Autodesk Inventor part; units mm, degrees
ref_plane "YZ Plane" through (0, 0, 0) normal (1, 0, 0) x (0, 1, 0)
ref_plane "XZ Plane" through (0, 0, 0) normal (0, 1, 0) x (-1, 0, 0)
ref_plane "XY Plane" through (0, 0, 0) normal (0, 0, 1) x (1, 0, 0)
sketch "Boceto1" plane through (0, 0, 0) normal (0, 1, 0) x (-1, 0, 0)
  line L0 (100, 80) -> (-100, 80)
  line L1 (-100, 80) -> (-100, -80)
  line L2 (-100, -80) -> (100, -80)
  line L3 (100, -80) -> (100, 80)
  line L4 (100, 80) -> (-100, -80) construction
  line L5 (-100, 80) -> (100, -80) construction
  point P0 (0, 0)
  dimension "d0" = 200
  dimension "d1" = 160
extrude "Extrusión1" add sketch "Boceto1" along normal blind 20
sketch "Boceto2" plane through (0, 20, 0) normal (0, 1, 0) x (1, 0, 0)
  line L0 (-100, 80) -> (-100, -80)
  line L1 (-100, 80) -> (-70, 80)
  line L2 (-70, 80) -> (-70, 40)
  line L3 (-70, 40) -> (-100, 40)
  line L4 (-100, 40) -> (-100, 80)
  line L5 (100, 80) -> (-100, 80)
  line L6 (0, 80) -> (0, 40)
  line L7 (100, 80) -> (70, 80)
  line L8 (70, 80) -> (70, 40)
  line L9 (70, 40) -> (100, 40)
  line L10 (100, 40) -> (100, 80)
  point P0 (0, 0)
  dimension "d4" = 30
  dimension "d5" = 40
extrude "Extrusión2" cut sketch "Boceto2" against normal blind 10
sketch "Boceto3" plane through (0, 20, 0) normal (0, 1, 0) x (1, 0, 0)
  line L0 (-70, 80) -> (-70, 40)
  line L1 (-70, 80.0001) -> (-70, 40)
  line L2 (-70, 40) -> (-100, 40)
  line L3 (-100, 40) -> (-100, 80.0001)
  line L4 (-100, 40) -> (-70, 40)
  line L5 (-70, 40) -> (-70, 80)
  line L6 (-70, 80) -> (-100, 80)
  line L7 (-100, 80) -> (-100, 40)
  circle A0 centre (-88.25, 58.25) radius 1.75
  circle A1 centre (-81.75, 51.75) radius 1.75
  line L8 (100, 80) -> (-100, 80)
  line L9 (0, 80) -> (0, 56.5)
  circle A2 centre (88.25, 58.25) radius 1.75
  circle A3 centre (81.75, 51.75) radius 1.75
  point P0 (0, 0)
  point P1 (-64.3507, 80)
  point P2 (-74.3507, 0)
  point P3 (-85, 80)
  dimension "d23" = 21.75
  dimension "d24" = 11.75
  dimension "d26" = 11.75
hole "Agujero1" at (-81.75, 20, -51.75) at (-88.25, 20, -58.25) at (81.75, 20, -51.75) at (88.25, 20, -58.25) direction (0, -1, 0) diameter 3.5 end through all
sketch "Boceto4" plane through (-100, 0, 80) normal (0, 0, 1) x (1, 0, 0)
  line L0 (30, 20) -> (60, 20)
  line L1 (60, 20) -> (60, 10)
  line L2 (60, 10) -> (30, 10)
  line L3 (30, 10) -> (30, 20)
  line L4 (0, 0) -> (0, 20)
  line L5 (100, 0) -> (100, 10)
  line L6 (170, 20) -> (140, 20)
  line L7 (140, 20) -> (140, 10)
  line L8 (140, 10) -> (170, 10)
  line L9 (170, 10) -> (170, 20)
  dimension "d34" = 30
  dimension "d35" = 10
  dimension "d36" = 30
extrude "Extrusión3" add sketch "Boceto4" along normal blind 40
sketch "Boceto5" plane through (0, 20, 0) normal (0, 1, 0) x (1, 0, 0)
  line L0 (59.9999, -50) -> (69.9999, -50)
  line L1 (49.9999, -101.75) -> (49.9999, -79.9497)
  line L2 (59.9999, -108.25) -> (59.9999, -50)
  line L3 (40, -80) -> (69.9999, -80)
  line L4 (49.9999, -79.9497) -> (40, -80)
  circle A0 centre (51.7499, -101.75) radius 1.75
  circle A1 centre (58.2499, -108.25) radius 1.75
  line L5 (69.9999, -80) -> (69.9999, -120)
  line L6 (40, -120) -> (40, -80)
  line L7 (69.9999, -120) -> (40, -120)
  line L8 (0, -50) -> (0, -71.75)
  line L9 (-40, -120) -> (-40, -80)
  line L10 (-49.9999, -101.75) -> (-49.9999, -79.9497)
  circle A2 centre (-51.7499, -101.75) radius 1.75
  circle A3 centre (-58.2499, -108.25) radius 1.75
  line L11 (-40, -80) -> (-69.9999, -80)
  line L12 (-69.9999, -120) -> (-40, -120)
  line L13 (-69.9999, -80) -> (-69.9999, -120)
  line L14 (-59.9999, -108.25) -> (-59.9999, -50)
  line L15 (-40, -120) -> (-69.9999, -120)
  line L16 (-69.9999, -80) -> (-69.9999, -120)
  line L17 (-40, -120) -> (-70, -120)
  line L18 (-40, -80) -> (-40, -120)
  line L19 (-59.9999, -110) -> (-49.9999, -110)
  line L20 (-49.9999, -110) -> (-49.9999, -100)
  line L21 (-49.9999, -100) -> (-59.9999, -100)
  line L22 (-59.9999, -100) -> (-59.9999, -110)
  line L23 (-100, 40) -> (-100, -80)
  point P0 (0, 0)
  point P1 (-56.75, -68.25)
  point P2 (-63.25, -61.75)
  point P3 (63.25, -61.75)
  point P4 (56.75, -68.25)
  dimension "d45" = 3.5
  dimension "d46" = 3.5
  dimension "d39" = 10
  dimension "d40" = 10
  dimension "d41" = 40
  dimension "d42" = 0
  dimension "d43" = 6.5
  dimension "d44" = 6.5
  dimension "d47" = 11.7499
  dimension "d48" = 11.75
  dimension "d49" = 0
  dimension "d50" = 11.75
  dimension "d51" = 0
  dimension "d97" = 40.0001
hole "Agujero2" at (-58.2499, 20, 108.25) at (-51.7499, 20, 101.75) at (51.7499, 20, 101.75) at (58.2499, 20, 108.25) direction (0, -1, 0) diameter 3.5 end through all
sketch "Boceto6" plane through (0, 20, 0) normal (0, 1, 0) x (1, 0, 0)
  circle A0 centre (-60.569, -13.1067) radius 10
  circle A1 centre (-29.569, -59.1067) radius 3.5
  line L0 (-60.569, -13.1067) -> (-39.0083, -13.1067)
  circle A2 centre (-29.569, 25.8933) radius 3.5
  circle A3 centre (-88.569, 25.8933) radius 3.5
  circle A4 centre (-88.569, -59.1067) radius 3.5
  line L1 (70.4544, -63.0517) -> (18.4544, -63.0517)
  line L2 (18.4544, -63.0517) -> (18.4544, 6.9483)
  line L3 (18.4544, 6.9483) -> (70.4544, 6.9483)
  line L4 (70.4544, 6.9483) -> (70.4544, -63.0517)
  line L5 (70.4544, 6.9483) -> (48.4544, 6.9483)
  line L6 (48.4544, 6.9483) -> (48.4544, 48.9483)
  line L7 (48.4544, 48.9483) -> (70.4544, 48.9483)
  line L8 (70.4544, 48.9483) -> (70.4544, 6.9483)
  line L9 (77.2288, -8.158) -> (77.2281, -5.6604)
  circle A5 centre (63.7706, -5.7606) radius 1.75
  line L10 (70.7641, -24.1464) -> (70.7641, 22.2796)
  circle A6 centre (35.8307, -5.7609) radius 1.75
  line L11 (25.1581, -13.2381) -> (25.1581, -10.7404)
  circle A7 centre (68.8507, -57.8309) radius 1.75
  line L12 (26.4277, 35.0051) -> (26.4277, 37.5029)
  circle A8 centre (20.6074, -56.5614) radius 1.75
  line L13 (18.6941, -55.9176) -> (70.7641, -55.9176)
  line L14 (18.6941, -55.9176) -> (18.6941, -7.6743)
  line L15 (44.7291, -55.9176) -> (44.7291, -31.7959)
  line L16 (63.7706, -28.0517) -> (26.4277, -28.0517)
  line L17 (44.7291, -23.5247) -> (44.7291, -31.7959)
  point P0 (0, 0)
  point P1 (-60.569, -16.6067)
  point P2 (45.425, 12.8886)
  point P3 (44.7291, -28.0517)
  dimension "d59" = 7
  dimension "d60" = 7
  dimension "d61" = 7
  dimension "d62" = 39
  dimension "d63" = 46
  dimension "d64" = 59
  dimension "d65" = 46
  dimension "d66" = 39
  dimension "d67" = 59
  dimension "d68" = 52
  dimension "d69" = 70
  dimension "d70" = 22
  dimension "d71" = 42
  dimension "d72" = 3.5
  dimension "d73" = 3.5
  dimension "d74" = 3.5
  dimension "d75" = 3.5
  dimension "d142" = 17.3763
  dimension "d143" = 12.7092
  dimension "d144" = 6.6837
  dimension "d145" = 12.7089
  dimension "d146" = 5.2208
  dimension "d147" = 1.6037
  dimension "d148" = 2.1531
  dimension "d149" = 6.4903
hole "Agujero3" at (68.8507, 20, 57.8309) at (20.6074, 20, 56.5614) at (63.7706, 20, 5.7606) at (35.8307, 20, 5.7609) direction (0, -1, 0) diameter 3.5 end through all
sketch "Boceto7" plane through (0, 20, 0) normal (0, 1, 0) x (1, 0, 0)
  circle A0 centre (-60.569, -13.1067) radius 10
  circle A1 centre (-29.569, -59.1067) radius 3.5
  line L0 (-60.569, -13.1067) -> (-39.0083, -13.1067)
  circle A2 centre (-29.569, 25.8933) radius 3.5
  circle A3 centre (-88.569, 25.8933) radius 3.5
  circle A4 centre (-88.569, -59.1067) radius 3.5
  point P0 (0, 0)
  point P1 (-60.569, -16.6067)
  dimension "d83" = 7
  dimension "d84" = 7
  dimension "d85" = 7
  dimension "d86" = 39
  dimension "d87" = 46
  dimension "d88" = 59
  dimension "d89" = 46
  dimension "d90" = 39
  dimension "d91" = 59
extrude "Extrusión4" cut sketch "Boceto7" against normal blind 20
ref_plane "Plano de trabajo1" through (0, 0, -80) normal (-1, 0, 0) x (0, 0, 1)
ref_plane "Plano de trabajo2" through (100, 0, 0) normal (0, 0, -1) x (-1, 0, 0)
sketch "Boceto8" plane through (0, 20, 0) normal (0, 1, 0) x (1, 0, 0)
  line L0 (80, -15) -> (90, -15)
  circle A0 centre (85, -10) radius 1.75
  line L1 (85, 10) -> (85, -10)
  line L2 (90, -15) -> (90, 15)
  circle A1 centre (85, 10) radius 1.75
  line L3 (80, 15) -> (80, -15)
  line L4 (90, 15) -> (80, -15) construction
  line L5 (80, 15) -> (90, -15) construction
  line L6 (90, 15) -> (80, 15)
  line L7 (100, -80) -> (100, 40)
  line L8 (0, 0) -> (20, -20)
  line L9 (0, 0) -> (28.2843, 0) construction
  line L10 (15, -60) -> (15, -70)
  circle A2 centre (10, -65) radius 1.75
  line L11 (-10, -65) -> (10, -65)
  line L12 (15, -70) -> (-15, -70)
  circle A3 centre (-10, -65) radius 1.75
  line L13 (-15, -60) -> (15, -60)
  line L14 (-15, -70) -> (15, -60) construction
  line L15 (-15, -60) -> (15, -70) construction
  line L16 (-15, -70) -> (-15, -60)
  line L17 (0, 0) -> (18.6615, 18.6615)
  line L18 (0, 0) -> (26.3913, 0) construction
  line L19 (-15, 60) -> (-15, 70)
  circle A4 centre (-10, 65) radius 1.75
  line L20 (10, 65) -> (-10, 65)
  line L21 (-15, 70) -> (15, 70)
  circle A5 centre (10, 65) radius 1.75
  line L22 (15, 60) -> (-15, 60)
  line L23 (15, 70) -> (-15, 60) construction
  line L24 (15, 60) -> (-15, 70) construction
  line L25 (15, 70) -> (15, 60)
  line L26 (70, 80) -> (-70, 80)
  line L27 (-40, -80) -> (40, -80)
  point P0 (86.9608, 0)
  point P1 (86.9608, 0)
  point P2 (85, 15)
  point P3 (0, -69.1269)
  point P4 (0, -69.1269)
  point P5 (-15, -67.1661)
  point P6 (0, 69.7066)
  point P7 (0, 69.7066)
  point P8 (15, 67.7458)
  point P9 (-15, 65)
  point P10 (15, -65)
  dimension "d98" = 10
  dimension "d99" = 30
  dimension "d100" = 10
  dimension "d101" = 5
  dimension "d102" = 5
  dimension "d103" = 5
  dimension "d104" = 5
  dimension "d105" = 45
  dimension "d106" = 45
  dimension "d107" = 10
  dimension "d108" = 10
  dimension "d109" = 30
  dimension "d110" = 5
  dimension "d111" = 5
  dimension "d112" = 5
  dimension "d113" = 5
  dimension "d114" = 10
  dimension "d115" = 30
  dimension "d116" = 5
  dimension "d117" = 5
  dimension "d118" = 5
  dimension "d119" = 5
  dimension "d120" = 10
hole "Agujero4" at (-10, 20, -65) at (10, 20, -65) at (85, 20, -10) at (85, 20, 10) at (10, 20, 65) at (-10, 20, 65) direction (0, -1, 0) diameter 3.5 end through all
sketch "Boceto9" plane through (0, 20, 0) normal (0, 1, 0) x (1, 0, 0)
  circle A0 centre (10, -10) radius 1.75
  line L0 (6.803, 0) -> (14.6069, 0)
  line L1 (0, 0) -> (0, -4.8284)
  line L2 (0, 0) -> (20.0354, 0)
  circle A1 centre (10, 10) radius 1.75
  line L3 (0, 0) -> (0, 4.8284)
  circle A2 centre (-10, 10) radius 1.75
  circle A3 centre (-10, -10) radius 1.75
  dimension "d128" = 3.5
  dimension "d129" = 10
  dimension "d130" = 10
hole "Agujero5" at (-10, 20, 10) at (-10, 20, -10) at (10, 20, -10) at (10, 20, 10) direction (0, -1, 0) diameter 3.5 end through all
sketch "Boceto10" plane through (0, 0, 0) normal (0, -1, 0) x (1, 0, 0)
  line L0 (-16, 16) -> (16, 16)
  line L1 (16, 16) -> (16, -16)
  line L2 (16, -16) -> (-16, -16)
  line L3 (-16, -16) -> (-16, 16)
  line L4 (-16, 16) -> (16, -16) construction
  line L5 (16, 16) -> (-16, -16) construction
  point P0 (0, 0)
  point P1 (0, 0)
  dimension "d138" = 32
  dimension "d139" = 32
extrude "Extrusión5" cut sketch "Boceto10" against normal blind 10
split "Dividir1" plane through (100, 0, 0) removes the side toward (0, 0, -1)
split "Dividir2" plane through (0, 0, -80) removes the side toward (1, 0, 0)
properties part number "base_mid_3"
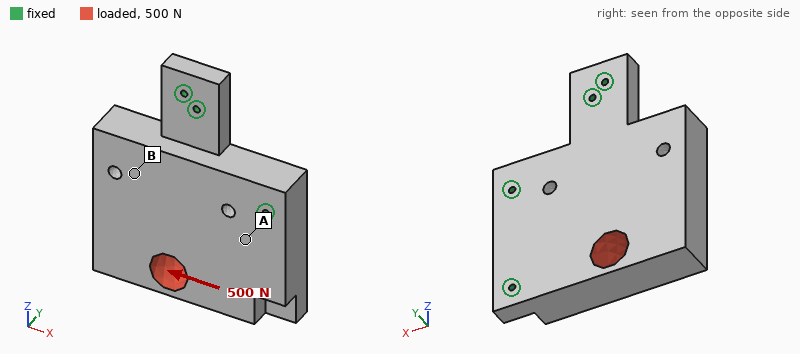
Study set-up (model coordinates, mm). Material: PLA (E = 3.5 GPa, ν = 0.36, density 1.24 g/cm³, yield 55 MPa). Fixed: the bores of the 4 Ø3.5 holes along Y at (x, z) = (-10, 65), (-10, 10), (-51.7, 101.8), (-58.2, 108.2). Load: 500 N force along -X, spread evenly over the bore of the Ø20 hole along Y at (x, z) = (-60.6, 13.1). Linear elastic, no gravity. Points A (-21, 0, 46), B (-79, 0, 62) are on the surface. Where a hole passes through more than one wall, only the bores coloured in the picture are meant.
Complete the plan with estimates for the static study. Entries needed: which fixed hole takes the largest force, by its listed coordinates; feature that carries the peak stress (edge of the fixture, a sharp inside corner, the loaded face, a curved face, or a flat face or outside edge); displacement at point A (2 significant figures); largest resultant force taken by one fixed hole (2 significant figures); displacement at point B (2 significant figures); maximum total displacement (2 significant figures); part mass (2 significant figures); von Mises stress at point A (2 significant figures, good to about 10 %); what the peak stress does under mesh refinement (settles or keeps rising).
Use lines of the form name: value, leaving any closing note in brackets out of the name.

which fixed hole takes the largest force, by its listed coordinates: (-10, 10)
feature that carries the peak stress: edge of the fixture
displacement at point A: 8.5 µm
largest resultant force taken by one fixed hole: 350 N
displacement at point B: 14 µm
maximum total displacement: 44 µm
part mass: 200 g
von Mises stress at point A: 0.61 MPa
what the peak stress does under mesh refinement: keeps rising
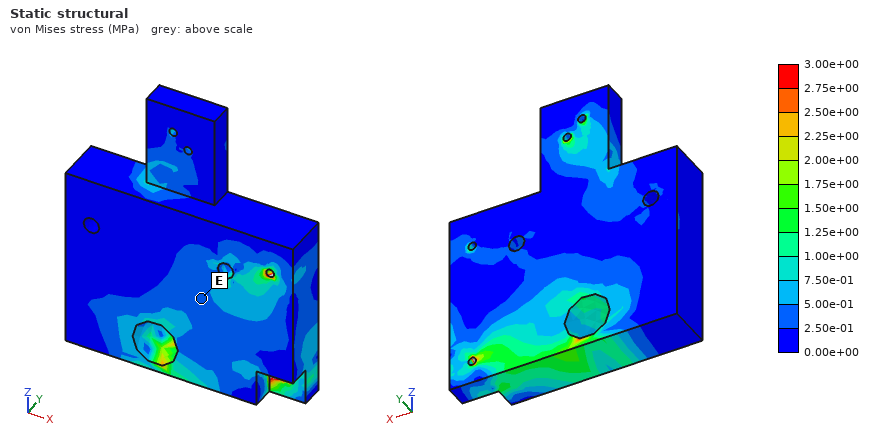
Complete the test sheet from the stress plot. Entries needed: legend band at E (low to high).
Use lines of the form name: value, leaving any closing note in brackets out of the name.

legend band at E: 2.50e-01 to 5.00e-01 MPa
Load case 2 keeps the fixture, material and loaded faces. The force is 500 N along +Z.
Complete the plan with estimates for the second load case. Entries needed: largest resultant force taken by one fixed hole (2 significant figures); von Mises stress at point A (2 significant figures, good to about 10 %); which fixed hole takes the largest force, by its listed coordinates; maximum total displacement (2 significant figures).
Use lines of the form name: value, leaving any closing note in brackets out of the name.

largest resultant force taken by one fixed hole: 220 N
von Mises stress at point A: 0.33 MPa
which fixed hole takes the largest force, by its listed coordinates: (-10, 10)
maximum total displacement: 32 µm
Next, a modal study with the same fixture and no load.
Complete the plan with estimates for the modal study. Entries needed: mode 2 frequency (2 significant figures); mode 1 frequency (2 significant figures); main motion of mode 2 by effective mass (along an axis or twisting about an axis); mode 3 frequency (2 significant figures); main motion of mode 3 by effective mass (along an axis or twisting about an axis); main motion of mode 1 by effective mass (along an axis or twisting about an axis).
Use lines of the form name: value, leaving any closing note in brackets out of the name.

mode 2 frequency: 1700 Hz
mode 1 frequency: 550 Hz
main motion of mode 2 by effective mass: twisting about X
mode 3 frequency: 2100 Hz
main motion of mode 3 by effective mass: along Z
main motion of mode 1 by effective mass: along Y
